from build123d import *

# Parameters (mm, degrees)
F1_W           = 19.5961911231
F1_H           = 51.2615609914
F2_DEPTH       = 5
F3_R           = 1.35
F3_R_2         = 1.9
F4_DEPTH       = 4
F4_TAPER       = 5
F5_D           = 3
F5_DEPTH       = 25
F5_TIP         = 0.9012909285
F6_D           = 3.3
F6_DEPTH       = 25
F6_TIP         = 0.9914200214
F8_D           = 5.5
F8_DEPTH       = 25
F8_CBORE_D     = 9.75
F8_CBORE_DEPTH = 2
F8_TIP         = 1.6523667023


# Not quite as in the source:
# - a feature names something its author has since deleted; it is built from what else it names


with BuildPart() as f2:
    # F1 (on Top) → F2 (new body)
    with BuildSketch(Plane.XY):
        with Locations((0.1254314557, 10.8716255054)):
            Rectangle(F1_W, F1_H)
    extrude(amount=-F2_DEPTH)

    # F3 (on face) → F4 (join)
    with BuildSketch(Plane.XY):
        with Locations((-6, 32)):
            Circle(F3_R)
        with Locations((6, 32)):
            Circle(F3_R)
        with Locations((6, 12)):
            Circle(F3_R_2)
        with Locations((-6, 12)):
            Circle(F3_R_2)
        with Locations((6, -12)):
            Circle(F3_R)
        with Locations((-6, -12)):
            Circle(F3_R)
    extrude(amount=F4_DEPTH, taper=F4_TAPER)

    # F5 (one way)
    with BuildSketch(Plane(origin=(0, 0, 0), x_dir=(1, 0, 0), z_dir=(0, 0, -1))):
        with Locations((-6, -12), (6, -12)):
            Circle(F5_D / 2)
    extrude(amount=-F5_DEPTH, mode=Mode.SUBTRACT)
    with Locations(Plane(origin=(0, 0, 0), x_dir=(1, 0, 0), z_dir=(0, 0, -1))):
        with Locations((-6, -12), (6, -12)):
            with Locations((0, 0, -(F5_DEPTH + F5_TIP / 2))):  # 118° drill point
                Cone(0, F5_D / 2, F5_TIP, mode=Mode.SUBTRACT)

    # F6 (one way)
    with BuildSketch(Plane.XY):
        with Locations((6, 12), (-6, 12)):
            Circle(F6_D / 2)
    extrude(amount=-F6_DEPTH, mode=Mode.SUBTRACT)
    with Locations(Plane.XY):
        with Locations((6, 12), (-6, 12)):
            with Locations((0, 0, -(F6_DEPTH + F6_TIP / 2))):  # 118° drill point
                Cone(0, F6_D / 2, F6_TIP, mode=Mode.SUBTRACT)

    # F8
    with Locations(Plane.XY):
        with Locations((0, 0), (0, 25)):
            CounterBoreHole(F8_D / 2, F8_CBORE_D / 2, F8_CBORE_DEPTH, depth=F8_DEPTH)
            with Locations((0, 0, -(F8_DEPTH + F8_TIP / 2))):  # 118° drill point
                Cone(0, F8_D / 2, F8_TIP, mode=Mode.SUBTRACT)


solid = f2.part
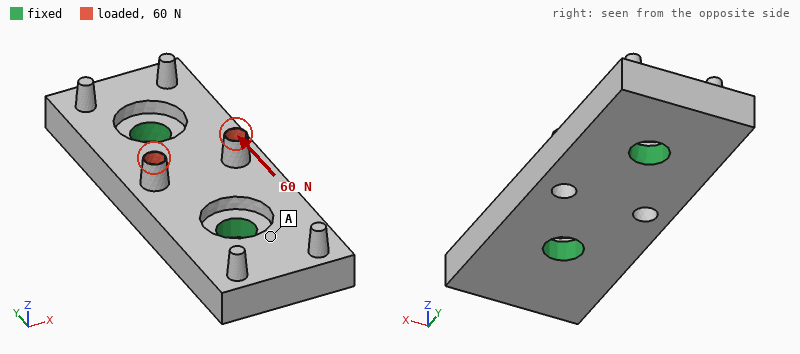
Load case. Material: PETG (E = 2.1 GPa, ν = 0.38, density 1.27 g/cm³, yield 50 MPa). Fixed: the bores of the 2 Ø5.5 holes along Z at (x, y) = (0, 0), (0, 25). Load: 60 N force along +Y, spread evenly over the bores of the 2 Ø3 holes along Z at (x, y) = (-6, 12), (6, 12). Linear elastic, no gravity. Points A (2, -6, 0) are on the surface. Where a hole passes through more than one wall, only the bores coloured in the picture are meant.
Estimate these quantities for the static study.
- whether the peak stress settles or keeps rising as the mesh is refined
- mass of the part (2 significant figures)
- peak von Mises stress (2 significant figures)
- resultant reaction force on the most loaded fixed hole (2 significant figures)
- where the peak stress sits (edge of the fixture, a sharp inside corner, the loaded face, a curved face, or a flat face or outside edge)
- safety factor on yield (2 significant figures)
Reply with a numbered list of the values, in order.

1. settles
2. 5.8 g
3. 27 MPa
4. 34 N
5. the loaded face
6. 1.9
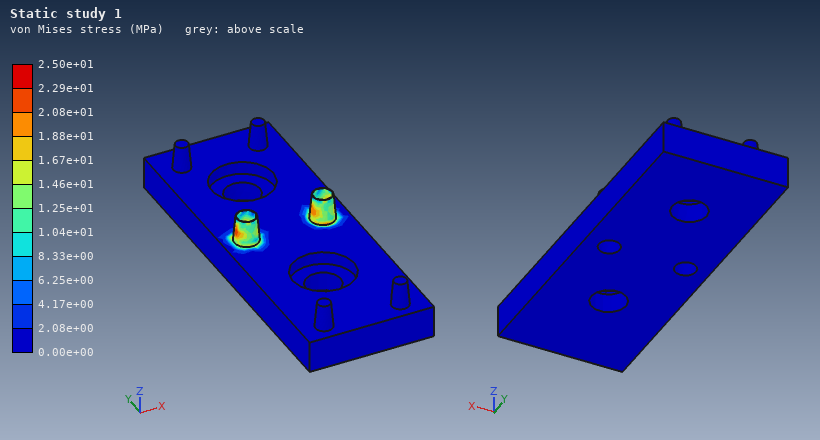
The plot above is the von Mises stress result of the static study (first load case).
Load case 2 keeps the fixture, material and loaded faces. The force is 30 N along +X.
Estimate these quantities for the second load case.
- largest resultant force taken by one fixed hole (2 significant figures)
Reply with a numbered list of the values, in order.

1. 16 N
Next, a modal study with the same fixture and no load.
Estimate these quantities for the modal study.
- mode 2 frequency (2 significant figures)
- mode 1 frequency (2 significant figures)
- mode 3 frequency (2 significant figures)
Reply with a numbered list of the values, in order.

1. 4500 Hz
2. 3500 Hz
3. 5300 Hz
